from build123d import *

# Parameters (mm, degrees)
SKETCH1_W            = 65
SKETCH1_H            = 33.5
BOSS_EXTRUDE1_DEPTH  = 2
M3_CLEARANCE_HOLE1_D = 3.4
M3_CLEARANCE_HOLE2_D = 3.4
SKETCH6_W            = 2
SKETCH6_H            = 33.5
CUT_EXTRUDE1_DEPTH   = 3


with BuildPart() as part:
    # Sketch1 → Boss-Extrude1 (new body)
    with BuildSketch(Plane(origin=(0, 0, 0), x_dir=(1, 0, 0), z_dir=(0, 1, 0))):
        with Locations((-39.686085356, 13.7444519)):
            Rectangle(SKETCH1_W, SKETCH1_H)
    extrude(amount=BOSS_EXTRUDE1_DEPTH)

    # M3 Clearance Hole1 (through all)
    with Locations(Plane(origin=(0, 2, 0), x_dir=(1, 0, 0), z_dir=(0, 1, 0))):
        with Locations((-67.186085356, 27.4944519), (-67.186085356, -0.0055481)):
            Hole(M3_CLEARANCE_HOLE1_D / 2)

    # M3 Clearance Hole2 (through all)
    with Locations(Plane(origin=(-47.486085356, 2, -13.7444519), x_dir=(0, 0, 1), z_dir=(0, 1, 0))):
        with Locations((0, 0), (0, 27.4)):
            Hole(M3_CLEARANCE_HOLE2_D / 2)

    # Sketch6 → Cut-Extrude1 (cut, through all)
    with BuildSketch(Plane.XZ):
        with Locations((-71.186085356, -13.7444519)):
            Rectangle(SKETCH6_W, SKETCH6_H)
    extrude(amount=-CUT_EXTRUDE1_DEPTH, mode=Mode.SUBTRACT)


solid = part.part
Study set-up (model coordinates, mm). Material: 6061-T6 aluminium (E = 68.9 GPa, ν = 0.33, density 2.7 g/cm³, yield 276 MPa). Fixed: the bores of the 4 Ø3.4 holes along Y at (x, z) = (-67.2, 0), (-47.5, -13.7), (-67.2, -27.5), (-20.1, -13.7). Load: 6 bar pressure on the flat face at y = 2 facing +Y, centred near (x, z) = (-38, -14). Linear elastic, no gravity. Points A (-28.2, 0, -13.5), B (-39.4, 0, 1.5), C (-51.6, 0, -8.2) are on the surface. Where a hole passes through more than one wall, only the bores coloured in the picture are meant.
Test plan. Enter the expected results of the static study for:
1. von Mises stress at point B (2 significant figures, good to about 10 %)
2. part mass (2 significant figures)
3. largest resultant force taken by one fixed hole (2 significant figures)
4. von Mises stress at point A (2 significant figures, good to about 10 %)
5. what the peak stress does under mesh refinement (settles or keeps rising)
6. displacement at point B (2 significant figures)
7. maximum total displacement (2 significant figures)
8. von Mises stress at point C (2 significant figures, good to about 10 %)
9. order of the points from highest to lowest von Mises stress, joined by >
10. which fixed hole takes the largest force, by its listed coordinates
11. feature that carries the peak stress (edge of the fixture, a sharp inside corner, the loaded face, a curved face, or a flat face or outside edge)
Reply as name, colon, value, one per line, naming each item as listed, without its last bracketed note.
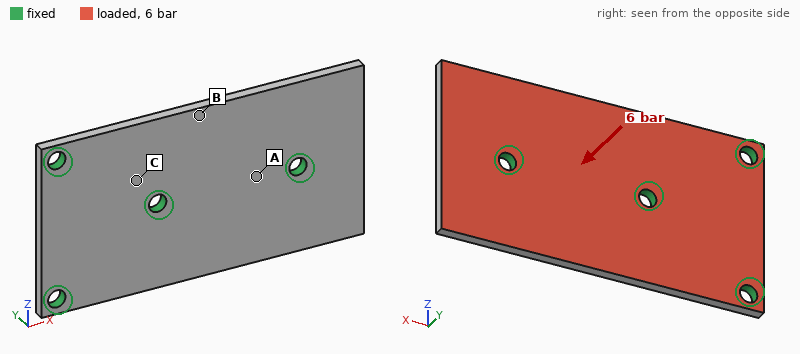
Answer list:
von Mises stress at point B: 18 MPa
part mass: 11 g
largest resultant force taken by one fixed hole: 540 N
von Mises stress at point A: 68 MPa
what the peak stress does under mesh refinement: keeps rising
displacement at point B: 0.089 mm
maximum total displacement: 0.12 mm
von Mises stress at point C: 42 MPa
order of the points from highest to lowest von Mises stress, joined by >: A > C > B
which fixed hole takes the largest force, by its listed coordinates: (-20.1, -13.7)
feature that carries the peak stress: edge of the fixture
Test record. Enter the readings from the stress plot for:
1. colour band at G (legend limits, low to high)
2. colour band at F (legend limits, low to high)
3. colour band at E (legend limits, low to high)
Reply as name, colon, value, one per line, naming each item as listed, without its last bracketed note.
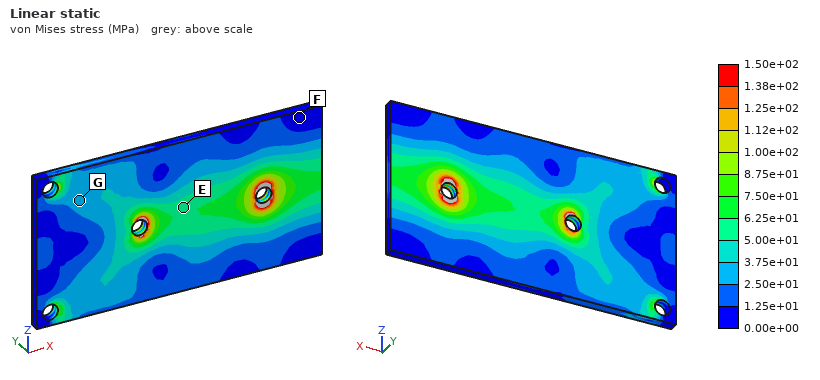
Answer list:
colour band at G: 2.50e+01 to 3.75e+01 MPa
colour band at F: 0.00e+00 to 1.25e+01 MPa
colour band at E: 5.00e+01 to 6.25e+01 MPa
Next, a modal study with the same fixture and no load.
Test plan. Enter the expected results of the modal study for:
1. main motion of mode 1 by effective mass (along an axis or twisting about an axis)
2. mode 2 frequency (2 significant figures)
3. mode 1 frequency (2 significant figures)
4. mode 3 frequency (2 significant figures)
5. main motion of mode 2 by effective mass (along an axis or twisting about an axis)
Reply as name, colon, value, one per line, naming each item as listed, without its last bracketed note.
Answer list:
main motion of mode 1 by effective mass: twisting about X
mode 2 frequency: 6400 Hz
mode 1 frequency: 5000 Hz
mode 3 frequency: 7100 Hz
main motion of mode 2 by effective mass: along Y
